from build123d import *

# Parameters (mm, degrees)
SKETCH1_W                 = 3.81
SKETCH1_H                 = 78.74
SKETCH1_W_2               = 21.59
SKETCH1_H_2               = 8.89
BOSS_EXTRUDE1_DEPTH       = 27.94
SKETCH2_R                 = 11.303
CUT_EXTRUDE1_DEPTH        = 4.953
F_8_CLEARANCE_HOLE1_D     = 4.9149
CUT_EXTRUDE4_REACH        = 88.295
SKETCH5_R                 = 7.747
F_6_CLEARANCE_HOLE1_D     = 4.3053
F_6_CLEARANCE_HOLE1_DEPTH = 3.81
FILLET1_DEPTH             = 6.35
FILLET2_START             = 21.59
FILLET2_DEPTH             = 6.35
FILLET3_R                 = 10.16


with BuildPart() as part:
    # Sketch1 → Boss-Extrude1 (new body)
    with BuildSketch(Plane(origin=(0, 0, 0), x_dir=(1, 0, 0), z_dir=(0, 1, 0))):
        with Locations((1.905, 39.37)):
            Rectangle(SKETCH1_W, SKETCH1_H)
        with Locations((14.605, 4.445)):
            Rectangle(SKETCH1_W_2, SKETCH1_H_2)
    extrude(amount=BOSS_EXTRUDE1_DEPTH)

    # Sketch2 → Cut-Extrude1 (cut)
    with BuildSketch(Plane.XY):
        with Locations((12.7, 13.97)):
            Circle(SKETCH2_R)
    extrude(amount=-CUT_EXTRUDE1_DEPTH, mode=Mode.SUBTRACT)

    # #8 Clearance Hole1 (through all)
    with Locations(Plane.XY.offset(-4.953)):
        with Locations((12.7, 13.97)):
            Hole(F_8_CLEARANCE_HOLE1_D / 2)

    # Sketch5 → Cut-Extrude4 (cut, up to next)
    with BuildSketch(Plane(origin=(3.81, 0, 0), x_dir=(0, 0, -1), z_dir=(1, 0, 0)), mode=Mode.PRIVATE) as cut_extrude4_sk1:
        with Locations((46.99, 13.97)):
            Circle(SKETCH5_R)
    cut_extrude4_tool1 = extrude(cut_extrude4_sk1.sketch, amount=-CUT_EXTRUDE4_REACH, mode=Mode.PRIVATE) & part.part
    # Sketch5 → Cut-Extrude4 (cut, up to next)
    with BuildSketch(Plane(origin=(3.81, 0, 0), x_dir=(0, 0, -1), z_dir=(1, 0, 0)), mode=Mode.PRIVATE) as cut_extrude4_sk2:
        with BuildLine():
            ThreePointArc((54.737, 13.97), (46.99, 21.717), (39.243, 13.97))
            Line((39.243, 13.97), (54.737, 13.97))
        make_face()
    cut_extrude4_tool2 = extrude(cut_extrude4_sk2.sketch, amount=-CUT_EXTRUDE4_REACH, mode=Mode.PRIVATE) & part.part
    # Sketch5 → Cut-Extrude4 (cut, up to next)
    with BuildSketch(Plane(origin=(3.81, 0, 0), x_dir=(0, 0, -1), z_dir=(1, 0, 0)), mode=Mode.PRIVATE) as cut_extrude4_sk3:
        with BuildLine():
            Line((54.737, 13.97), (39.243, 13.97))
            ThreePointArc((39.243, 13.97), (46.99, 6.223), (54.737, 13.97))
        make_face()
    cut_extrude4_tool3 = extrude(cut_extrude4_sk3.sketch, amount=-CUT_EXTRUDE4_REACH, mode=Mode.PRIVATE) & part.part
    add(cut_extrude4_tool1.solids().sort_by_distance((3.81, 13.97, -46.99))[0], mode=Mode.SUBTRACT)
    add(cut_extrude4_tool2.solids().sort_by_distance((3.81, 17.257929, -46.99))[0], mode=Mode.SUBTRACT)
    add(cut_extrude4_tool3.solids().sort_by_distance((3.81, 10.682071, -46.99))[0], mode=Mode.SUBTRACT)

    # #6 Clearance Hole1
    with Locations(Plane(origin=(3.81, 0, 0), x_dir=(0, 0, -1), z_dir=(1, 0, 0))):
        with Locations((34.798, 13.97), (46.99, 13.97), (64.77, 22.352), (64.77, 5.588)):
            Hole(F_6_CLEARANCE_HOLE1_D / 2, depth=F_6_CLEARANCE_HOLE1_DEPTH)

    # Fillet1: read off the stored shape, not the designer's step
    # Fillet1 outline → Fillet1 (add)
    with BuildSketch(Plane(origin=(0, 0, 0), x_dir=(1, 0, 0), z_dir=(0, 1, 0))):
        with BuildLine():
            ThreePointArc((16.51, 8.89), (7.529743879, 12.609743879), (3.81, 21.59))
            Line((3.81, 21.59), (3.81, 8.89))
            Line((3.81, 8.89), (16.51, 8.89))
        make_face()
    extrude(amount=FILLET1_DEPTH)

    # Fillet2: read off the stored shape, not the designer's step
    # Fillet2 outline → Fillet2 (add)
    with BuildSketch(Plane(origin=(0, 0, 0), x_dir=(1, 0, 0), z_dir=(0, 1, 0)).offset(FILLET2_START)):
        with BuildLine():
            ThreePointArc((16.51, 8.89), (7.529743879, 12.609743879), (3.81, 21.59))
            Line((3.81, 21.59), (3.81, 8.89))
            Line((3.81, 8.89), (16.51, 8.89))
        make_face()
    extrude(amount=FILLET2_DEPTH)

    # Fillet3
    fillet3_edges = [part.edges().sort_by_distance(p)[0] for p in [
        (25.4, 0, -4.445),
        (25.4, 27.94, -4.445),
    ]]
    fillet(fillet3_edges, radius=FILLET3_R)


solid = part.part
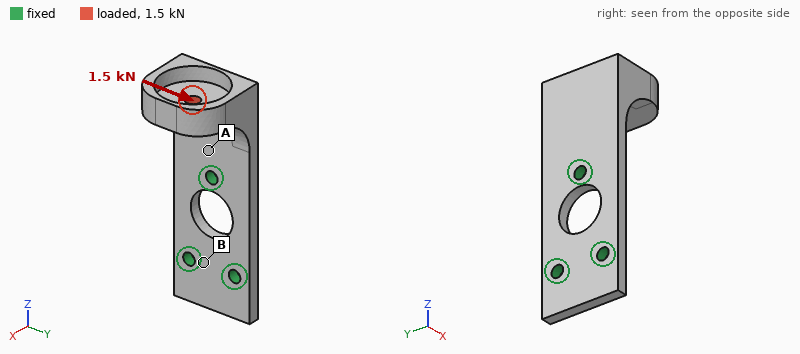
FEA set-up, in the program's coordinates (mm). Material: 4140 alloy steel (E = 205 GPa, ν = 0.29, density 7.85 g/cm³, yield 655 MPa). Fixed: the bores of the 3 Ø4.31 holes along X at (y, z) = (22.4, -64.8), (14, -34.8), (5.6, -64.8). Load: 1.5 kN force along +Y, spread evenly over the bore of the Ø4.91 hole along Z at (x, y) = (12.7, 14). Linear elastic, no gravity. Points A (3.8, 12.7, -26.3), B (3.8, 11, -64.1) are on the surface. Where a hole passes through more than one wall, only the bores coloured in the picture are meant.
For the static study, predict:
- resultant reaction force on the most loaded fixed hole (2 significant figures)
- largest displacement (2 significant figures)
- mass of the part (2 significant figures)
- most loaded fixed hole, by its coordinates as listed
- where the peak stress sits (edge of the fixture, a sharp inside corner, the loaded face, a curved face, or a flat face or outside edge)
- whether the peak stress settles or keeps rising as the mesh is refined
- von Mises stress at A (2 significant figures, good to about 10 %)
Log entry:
2.0 kN
0.21 mm
85 g
(14, -34.8)
edge of the fixture
keeps rising
220 MPa
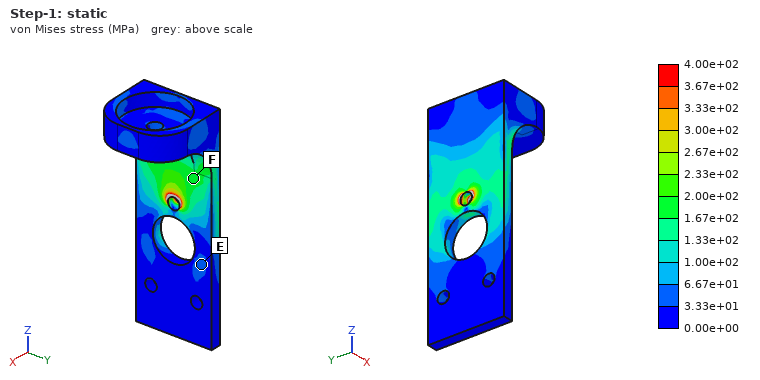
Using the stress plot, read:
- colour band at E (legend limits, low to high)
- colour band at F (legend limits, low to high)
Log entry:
3.33e+01 to 6.67e+01 MPa
1.67e+02 to 2.00e+02 MPa
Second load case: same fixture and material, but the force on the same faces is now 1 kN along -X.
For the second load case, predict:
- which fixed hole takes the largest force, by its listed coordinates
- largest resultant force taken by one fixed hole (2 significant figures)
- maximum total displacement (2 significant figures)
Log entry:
(14, -34.8)
1.3 kN
0.49 mm
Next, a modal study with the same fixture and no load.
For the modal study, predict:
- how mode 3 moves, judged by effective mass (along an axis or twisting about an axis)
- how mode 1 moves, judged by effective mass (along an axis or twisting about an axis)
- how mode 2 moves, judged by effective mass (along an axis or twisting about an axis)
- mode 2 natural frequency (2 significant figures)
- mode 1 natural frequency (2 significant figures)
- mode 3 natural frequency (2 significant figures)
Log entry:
along Y
along X
along Y
2500 Hz
1300 Hz
6400 Hz
